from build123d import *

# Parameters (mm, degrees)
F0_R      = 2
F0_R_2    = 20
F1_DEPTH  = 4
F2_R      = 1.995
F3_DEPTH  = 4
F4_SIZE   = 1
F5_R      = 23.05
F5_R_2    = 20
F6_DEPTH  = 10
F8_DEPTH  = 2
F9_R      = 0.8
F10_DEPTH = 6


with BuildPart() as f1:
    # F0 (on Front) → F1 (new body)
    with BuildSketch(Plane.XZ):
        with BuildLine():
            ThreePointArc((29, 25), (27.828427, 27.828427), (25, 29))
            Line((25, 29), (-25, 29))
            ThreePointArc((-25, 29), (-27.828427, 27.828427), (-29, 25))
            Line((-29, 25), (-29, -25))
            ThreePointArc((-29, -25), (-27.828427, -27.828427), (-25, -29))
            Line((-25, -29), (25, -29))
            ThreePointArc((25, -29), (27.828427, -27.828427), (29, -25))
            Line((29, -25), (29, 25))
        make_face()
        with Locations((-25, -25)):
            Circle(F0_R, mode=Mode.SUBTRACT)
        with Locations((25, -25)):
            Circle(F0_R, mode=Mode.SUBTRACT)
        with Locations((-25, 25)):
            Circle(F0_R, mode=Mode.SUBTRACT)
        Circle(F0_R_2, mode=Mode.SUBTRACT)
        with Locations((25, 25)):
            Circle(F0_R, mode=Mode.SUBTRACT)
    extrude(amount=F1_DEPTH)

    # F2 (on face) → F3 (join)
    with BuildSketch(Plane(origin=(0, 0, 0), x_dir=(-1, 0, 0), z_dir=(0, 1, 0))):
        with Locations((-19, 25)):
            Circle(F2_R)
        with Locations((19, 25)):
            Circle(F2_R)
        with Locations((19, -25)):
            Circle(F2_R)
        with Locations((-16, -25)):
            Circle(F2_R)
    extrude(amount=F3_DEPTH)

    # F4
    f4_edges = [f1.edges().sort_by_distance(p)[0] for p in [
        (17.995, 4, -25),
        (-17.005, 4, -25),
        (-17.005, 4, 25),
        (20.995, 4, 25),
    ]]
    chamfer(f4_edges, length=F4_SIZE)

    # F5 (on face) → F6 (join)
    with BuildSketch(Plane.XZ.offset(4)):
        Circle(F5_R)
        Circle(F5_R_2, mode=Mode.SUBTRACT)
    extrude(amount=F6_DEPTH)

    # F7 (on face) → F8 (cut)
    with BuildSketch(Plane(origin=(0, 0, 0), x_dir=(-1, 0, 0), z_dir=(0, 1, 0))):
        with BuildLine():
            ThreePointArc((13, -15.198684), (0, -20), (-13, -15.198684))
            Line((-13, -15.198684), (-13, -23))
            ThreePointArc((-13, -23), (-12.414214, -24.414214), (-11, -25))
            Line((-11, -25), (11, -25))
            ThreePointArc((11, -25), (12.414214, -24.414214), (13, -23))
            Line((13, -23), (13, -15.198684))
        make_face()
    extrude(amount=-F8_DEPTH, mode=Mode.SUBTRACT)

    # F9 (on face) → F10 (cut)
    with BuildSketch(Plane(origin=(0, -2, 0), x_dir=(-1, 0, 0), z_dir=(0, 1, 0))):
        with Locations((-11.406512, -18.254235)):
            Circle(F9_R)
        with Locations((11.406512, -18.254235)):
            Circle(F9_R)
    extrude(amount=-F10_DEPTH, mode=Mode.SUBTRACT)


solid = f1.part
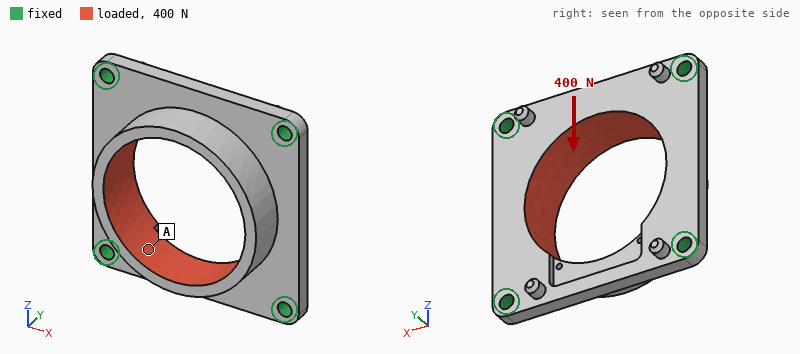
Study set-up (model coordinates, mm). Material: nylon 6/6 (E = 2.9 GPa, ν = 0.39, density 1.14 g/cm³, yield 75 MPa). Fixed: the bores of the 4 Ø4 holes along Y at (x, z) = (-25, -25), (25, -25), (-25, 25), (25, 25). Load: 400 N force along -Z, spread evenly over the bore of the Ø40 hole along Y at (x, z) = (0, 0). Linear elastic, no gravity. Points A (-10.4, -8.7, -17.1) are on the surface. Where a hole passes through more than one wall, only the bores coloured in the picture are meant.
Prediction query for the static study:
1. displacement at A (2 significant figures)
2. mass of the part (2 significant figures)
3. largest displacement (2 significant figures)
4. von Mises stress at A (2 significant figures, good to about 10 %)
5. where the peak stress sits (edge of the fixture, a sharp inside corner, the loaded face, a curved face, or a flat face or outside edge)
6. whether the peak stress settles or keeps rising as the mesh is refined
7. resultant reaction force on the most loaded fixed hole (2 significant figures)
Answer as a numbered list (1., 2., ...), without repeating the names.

1. 45 µm
2. 14 g
3. 85 µm
4. 1.6 MPa
5. edge of the fixture
6. keeps rising
7. 110 N
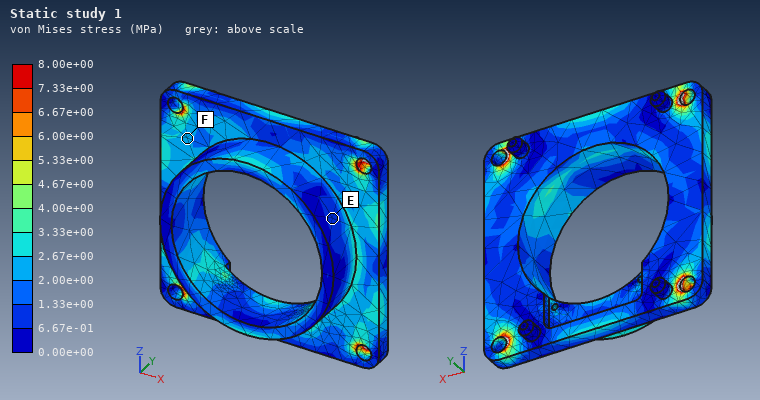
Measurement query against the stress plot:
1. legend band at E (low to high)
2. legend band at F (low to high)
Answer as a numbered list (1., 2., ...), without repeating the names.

1. 6.67e-01 to 1.33e+00 MPa
2. 2.00e+00 to 2.67e+00 MPa
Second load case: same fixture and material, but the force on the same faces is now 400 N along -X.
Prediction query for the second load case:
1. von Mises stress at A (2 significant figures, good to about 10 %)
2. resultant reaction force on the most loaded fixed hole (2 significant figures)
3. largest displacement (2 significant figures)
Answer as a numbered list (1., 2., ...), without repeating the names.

1. 2.8 MPa
2. 110 N
3. 82 µm
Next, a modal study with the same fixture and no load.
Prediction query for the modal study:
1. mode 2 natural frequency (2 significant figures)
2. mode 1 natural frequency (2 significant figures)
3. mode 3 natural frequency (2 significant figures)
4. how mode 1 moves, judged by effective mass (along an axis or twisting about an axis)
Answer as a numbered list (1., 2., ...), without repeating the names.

1. 2900 Hz
2. 2600 Hz
3. 3000 Hz
4. along Y
